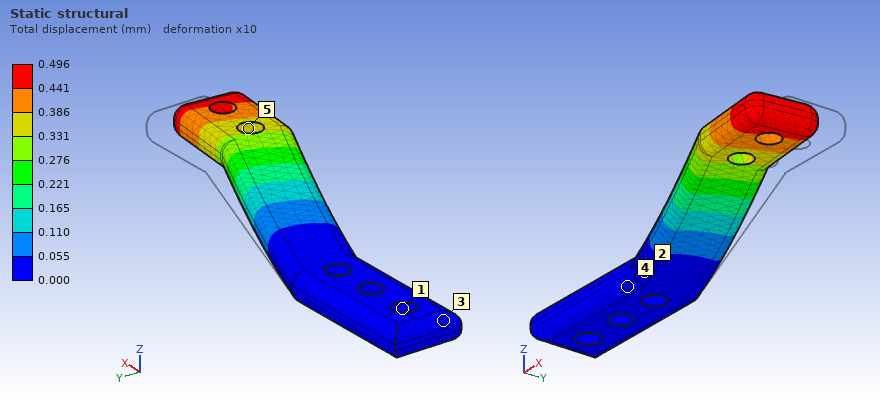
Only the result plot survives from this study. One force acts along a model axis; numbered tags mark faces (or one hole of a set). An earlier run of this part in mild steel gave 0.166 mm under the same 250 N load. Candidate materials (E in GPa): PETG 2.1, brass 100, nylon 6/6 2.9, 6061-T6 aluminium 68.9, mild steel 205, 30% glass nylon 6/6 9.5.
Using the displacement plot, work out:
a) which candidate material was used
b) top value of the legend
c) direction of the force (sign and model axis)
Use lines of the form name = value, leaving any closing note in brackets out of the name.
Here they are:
which candidate material was used = 6061-T6 aluminium
top value of the legend = 0.496 mm
direction of the force = -Y
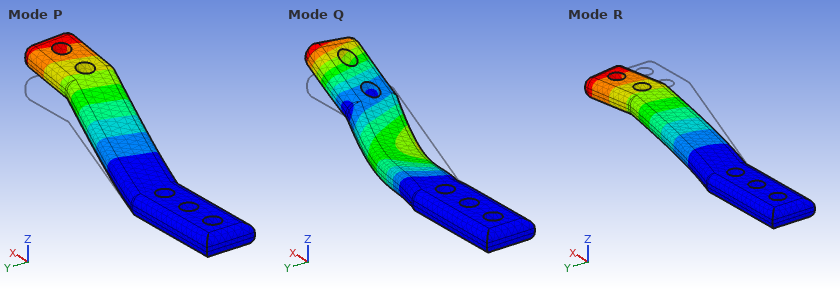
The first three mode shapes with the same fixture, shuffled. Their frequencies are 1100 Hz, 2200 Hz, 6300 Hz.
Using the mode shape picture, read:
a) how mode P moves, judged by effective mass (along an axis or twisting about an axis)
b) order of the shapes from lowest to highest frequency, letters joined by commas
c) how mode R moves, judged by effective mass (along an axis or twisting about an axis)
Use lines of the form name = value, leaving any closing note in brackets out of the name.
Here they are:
how mode P moves, judged by effective mass = along Z
order of the shapes from lowest to highest frequency, letters joined by commas = P, R, Q
how mode R moves, judged by effective mass = along Y
